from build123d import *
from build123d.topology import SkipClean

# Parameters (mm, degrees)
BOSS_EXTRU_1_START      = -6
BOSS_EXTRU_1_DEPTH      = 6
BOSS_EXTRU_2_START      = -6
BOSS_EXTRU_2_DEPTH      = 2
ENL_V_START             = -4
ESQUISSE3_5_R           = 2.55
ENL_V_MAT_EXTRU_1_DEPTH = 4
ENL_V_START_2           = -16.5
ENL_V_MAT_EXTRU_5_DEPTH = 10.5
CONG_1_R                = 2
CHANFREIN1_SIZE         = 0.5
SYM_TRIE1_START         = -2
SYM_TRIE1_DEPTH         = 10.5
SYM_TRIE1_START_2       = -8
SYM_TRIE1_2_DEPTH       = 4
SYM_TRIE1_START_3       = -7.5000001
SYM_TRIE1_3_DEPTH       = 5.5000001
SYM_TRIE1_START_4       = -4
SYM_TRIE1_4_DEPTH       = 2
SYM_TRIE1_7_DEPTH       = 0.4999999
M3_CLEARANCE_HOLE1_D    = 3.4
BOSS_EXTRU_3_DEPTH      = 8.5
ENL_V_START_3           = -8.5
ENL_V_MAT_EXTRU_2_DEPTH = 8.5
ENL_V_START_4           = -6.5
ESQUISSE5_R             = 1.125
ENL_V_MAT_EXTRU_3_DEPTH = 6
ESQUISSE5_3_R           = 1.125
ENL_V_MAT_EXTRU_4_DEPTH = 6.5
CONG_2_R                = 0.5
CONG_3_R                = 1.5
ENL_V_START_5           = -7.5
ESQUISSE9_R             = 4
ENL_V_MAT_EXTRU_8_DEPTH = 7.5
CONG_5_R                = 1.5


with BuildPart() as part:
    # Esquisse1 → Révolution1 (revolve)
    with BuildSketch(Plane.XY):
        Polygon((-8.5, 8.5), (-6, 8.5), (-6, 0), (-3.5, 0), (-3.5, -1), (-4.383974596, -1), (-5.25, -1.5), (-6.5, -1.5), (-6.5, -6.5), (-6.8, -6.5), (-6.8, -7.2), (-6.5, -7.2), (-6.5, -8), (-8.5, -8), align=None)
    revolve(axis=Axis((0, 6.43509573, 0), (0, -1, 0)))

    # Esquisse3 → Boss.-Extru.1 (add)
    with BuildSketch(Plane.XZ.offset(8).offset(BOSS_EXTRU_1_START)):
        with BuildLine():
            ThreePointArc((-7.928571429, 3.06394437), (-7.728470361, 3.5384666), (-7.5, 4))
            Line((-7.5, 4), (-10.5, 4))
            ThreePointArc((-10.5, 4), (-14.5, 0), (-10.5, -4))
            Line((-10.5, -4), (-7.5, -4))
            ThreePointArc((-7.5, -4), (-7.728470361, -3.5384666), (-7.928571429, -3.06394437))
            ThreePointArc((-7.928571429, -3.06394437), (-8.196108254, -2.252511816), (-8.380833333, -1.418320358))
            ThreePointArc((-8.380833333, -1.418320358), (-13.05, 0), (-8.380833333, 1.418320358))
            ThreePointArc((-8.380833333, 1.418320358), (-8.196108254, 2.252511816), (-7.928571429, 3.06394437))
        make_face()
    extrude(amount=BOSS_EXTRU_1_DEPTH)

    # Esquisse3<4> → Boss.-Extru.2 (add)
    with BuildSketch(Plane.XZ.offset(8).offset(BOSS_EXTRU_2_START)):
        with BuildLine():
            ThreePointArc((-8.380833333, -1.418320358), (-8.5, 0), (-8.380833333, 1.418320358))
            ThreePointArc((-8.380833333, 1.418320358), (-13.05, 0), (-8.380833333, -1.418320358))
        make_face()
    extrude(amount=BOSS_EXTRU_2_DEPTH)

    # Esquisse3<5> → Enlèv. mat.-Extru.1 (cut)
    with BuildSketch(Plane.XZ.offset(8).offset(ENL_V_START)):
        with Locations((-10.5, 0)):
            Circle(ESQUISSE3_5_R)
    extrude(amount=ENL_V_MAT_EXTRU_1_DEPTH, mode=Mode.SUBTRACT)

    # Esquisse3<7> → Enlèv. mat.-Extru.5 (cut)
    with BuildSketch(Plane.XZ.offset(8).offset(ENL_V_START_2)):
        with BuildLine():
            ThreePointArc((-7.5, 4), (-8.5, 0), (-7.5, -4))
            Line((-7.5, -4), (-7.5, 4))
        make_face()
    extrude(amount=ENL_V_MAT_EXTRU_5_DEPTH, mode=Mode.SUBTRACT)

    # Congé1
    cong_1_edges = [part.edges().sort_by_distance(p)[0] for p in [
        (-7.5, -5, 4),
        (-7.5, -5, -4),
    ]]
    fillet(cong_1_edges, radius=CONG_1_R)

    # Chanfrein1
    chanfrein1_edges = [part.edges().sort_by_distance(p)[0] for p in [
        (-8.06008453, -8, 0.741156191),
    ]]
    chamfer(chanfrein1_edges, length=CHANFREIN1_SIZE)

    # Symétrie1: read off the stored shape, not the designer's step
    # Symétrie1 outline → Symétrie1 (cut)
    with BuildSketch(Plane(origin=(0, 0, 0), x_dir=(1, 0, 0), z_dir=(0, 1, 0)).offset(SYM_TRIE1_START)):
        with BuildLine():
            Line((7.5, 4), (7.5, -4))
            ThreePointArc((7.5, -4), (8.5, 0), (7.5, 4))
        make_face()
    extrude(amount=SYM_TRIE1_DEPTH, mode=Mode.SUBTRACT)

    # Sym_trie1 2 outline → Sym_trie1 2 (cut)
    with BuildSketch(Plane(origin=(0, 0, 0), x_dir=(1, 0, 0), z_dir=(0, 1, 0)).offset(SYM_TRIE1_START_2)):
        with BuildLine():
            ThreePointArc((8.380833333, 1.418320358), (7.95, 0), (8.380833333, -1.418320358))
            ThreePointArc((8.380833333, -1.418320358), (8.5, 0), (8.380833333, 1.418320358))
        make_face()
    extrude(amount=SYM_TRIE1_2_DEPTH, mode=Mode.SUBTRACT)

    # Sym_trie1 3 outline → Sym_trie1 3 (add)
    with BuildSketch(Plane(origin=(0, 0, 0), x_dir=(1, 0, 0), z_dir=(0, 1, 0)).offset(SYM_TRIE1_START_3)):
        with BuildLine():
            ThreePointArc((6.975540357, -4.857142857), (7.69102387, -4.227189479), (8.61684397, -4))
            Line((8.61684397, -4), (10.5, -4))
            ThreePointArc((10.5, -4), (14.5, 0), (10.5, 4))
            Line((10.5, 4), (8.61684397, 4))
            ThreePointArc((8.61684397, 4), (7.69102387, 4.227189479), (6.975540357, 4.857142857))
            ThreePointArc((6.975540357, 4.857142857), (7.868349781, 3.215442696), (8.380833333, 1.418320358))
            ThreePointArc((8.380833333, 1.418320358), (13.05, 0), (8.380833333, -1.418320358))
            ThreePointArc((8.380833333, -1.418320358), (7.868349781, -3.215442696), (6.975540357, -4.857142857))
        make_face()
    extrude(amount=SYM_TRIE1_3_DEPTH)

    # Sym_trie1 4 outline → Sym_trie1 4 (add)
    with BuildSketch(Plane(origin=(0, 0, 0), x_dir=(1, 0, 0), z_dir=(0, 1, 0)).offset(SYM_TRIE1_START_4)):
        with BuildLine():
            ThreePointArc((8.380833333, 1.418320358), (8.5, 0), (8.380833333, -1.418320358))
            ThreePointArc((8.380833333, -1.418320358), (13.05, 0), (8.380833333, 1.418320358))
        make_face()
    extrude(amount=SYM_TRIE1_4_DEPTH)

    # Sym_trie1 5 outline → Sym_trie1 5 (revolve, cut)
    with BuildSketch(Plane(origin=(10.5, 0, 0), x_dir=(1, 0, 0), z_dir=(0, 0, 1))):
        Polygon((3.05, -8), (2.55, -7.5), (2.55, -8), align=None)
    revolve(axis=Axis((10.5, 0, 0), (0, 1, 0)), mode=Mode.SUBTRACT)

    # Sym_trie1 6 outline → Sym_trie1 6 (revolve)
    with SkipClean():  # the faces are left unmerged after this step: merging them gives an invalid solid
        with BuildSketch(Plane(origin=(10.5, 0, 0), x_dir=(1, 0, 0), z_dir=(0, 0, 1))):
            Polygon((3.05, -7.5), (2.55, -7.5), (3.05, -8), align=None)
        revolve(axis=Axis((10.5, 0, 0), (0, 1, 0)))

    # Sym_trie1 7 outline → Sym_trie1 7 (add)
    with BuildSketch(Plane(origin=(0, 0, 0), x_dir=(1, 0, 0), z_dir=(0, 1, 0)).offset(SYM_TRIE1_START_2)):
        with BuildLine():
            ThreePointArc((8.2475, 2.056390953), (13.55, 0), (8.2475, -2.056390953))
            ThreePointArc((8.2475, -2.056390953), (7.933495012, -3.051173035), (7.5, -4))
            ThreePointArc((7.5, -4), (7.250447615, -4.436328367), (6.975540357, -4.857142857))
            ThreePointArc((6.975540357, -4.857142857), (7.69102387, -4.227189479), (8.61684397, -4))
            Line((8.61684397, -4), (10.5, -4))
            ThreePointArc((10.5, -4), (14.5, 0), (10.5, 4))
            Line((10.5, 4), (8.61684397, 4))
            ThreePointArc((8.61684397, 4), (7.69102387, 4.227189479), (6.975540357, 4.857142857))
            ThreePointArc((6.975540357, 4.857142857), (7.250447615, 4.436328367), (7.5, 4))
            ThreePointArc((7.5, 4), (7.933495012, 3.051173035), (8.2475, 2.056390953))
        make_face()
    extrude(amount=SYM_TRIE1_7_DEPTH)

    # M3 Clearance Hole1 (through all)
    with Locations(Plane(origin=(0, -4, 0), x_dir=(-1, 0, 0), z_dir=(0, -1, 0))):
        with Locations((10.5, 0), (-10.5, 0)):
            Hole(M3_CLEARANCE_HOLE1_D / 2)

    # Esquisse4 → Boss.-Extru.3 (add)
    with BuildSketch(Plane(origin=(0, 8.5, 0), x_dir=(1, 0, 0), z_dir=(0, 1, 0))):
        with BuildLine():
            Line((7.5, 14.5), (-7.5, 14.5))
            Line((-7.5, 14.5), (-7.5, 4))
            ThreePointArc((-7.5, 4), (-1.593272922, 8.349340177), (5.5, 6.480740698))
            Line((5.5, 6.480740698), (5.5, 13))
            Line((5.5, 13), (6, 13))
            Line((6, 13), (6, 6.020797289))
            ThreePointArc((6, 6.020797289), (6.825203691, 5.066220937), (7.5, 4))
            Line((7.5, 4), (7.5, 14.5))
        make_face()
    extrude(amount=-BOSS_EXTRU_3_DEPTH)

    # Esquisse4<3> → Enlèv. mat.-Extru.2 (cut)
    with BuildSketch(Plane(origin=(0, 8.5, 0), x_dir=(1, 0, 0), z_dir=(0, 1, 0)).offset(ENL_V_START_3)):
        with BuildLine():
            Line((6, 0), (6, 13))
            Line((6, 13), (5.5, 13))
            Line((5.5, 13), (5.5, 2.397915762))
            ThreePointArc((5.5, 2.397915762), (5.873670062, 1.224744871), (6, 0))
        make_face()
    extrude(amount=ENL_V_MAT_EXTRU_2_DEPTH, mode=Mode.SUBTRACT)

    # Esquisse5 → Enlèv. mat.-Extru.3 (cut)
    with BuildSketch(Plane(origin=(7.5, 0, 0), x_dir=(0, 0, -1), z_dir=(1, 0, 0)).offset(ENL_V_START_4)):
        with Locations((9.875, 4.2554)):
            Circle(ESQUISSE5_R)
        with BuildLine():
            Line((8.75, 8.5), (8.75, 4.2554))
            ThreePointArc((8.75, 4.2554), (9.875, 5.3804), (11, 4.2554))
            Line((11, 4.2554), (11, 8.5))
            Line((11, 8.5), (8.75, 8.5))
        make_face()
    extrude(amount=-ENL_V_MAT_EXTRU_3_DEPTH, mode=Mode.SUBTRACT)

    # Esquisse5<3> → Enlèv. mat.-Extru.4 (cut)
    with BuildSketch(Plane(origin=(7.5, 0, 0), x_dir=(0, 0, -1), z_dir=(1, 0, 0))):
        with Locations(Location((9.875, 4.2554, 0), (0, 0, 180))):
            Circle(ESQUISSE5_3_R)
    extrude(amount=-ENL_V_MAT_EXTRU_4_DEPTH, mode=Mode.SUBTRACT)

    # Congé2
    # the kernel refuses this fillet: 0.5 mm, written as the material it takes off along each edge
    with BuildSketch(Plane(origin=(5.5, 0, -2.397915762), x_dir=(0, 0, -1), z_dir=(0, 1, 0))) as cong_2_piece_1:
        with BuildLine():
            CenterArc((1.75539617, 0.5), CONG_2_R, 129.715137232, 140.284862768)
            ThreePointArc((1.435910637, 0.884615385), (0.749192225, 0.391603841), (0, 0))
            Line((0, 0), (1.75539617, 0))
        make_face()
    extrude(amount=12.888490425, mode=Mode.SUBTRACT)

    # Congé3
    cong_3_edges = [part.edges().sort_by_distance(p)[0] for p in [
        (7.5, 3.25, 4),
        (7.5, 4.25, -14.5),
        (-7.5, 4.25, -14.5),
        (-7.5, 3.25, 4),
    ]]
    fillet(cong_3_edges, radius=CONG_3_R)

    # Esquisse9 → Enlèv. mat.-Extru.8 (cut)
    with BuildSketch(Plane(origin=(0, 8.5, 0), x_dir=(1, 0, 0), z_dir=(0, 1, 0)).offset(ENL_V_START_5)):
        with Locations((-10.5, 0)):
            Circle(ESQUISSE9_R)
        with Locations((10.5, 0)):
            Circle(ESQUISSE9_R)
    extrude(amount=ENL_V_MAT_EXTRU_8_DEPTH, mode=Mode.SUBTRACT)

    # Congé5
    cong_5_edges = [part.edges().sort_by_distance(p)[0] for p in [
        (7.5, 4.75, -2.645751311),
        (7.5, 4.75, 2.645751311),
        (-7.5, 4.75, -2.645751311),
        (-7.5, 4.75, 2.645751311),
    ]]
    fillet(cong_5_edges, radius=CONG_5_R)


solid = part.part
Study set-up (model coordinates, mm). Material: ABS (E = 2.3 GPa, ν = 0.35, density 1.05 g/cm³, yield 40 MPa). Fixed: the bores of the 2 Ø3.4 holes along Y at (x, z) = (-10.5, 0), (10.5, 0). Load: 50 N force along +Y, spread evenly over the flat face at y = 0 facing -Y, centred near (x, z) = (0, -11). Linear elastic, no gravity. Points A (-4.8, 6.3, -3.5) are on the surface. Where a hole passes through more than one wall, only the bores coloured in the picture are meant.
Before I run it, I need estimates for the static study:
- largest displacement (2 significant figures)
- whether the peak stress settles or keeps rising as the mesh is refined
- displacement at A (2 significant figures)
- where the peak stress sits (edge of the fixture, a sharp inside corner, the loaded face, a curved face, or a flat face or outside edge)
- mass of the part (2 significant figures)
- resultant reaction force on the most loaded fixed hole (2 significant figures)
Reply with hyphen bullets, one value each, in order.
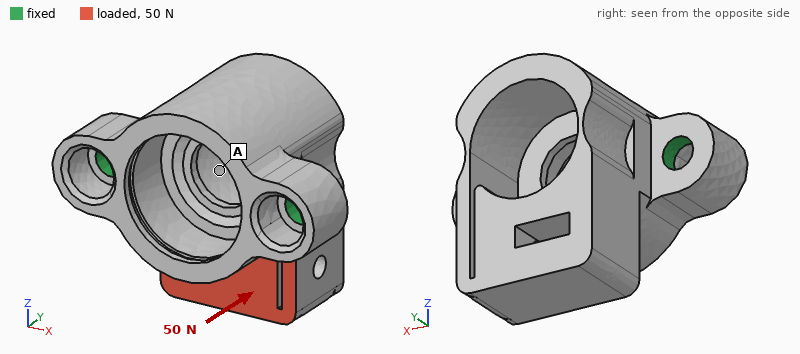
- 0.30 mm
- keeps rising
- 0.15 mm
- edge of the fixture
- 2.9 g
- 28 N
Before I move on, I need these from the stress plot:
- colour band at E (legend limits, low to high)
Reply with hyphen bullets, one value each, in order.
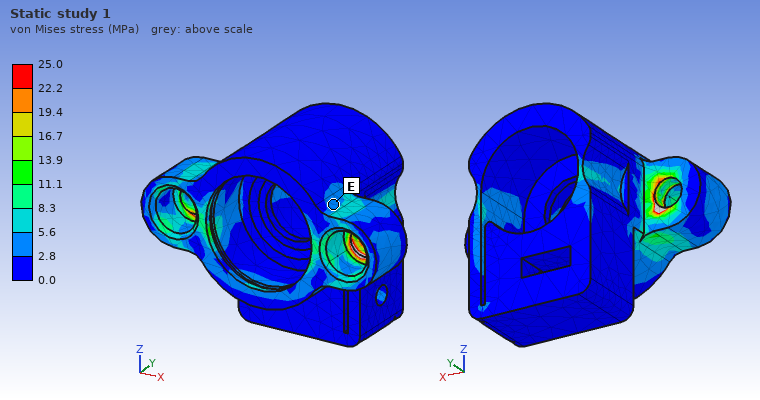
- 2.8 to 5.6 MPa
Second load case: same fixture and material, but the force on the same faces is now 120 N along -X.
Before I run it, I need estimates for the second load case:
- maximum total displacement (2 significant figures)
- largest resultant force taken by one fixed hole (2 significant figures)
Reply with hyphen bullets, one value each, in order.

- 0.11 mm
- 90 N
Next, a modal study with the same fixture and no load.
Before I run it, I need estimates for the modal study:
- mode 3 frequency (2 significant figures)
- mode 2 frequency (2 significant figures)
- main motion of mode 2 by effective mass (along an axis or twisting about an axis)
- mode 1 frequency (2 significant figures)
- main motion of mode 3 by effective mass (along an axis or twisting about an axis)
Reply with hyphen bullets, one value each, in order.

- 5900 Hz
- 5000 Hz
- along X
- 1900 Hz
- along Y
